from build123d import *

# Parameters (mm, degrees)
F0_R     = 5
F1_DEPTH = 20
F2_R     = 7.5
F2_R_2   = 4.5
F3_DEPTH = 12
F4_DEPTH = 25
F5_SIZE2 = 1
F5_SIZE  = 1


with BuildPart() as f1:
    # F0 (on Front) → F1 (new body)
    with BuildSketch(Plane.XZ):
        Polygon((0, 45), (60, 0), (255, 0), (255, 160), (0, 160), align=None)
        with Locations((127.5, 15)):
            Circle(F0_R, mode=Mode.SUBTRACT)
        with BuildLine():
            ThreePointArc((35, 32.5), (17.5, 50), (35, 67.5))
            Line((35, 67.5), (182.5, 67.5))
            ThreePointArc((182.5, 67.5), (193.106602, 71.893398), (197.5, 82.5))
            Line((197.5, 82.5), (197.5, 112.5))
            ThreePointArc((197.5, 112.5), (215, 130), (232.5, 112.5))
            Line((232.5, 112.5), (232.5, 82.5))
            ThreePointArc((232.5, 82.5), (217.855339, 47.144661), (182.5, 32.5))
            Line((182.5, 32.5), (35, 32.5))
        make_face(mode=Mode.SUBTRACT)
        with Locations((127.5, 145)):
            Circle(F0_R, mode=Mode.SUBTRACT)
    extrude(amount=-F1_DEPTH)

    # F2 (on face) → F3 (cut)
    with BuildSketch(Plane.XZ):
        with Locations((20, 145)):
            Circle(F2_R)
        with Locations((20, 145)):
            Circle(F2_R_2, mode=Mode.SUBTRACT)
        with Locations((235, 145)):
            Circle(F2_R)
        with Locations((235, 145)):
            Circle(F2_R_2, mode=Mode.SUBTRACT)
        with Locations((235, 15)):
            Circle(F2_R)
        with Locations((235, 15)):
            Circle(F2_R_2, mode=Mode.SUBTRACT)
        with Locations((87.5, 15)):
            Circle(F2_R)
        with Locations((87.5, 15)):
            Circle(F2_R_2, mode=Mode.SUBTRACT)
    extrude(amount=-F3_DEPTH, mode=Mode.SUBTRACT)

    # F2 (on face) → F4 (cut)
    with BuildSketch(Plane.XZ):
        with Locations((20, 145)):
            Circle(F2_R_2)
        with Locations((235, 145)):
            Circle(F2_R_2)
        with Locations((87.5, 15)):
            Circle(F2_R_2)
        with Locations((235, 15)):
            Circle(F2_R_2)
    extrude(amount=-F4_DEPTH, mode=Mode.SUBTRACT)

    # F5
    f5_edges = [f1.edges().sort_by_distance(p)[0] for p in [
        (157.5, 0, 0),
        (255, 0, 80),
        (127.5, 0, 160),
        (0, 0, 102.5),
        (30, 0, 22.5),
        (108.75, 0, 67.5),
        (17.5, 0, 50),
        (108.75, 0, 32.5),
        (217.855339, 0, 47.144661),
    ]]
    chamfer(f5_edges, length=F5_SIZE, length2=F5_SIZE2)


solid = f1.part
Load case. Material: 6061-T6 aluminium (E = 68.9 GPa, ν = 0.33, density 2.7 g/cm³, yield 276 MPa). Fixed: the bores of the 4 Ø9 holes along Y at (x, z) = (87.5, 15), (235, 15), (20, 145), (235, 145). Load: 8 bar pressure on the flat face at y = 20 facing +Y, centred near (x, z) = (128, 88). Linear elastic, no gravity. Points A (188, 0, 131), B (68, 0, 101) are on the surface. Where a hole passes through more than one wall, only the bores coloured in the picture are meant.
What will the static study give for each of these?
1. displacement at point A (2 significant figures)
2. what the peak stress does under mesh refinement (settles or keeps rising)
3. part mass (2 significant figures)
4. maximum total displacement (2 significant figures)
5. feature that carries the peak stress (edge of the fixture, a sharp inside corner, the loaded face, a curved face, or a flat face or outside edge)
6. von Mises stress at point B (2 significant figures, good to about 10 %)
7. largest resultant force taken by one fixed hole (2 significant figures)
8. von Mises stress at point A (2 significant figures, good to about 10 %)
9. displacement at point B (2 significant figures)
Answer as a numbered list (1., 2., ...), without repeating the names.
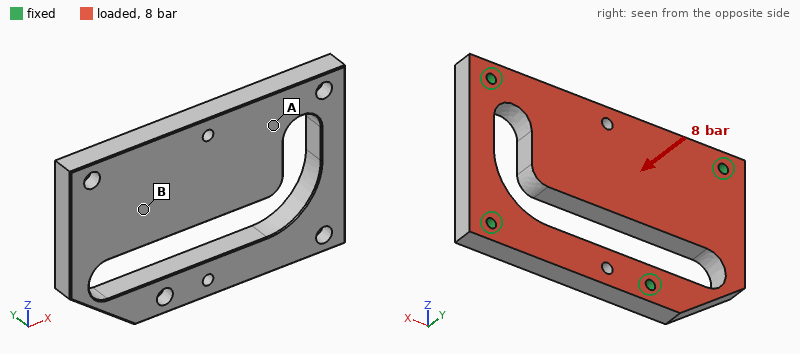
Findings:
1. 0.24 mm
2. keeps rising
3. 1.6 kg
4. 0.65 mm
5. edge of the fixture
6. 20 MPa
7. 10 kN
8. 58 MPa
9. 0.34 mm
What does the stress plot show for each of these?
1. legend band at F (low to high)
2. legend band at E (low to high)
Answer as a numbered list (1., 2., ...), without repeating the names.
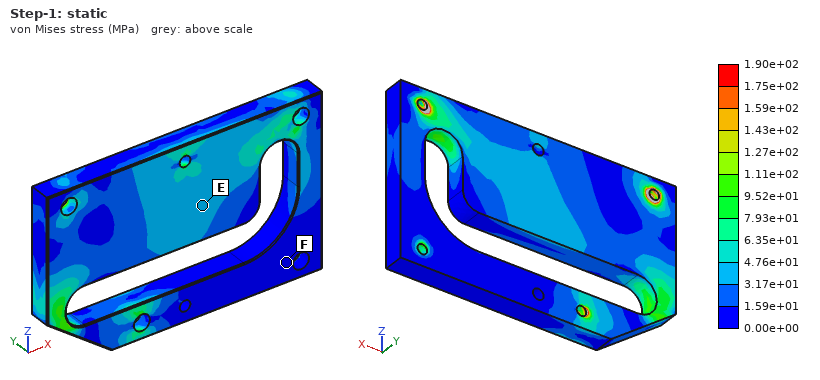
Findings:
1. 0.00e+00 to 1.59e+01 MPa
2. 3.17e+01 to 4.76e+01 MPa
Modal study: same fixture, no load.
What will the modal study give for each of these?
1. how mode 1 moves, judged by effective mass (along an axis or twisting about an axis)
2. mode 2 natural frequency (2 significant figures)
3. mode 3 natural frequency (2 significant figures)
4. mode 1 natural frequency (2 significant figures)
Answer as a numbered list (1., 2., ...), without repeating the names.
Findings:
1. along Y
2. 1900 Hz
3. 2500 Hz
4. 980 Hz
